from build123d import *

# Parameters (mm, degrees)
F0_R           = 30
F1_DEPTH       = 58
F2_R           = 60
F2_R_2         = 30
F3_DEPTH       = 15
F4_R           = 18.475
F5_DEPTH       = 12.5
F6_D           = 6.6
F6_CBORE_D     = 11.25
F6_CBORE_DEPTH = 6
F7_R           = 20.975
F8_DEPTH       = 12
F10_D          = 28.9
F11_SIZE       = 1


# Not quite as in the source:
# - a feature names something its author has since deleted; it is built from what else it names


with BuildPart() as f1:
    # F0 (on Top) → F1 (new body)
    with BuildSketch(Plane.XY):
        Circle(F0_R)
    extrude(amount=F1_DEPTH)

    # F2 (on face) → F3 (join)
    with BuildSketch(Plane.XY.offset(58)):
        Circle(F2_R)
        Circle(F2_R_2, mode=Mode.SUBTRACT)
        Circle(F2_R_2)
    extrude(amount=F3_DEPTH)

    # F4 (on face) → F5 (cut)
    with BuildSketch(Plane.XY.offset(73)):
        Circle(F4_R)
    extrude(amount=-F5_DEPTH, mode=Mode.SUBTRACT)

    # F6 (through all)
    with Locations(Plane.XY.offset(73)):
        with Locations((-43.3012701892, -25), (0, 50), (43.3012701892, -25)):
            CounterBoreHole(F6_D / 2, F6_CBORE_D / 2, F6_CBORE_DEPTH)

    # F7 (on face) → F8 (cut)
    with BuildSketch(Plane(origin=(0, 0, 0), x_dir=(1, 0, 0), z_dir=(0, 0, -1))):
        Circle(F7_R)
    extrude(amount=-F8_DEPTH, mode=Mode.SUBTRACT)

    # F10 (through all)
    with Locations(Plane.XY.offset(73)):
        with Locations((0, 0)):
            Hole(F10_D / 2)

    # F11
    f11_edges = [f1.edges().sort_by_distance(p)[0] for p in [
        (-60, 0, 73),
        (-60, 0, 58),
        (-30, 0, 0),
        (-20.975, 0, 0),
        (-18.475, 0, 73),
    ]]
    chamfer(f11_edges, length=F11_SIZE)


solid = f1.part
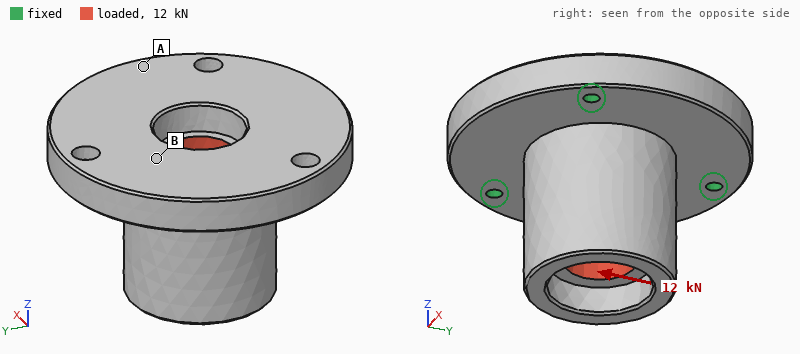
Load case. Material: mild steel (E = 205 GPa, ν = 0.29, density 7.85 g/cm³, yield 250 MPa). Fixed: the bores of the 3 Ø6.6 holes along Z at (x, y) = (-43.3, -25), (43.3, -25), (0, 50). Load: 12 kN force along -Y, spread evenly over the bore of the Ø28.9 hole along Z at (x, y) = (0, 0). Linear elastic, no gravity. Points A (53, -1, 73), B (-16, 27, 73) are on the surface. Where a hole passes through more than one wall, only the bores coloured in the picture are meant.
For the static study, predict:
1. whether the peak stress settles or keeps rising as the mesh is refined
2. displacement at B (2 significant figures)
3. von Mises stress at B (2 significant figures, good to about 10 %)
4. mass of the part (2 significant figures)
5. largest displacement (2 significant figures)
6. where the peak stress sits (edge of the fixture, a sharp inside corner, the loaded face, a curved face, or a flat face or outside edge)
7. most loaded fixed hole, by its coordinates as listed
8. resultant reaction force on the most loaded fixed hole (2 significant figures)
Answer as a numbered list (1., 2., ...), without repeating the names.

1. keeps rising
2. 5.5 µm
3. 18 MPa
4. 2.1 kg
5. 23 µm
6. edge of the fixture
7. (0, 50)
8. 5.6 kN
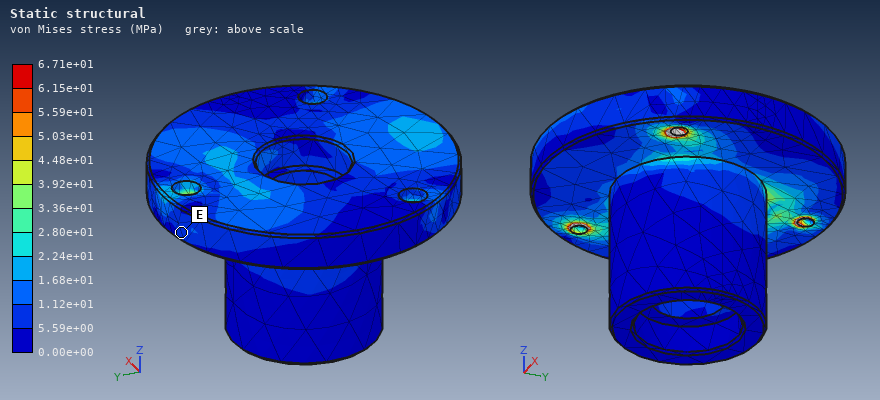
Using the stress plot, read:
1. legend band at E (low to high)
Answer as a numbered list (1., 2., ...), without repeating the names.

1. 5.59e+00 to 1.12e+01 MPa
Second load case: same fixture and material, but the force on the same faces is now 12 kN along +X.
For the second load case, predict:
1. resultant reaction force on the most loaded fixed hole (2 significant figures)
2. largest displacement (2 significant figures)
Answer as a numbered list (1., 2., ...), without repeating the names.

1. 5.3 kN
2. 23 µm
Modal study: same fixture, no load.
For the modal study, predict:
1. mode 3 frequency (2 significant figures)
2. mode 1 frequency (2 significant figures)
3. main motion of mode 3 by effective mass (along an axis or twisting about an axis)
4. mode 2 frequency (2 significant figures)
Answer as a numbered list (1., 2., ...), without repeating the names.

1. 4600 Hz
2. 3600 Hz
3. along Z
4. 3600 Hz
